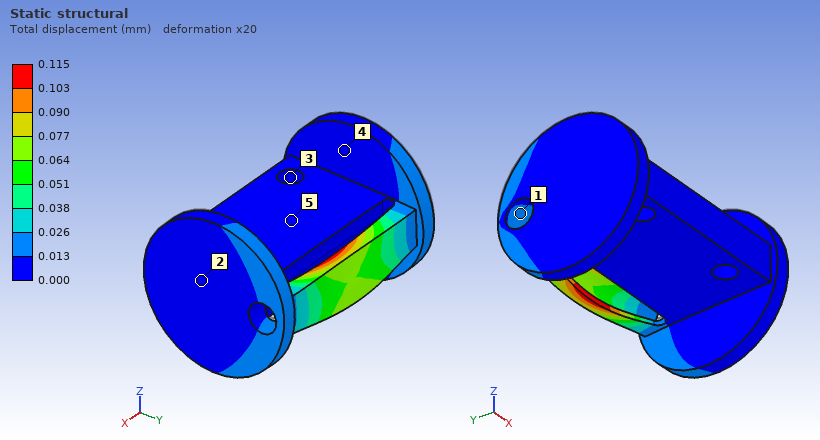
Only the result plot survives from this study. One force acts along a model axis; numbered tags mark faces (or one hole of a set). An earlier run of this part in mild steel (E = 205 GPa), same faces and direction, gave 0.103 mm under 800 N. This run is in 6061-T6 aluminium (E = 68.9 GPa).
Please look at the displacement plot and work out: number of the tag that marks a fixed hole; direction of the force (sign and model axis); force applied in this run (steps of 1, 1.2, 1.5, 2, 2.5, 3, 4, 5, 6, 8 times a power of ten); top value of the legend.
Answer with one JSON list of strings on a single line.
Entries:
["3", "-Z", "300 N", "0.115 mm"]
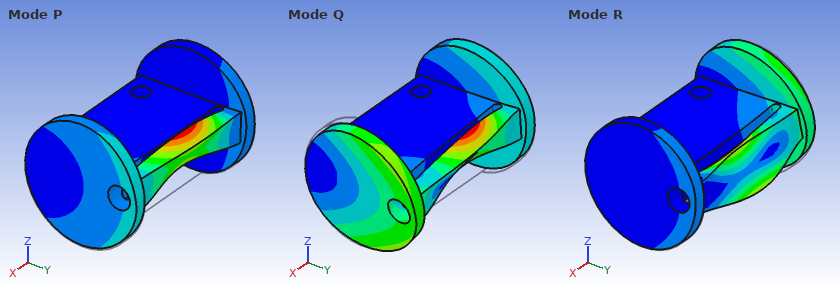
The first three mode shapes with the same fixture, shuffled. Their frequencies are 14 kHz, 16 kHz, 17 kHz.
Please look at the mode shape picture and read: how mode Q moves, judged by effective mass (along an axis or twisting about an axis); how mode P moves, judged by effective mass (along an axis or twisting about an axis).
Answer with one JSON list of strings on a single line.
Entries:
["twisting about Y", "along Z"]
